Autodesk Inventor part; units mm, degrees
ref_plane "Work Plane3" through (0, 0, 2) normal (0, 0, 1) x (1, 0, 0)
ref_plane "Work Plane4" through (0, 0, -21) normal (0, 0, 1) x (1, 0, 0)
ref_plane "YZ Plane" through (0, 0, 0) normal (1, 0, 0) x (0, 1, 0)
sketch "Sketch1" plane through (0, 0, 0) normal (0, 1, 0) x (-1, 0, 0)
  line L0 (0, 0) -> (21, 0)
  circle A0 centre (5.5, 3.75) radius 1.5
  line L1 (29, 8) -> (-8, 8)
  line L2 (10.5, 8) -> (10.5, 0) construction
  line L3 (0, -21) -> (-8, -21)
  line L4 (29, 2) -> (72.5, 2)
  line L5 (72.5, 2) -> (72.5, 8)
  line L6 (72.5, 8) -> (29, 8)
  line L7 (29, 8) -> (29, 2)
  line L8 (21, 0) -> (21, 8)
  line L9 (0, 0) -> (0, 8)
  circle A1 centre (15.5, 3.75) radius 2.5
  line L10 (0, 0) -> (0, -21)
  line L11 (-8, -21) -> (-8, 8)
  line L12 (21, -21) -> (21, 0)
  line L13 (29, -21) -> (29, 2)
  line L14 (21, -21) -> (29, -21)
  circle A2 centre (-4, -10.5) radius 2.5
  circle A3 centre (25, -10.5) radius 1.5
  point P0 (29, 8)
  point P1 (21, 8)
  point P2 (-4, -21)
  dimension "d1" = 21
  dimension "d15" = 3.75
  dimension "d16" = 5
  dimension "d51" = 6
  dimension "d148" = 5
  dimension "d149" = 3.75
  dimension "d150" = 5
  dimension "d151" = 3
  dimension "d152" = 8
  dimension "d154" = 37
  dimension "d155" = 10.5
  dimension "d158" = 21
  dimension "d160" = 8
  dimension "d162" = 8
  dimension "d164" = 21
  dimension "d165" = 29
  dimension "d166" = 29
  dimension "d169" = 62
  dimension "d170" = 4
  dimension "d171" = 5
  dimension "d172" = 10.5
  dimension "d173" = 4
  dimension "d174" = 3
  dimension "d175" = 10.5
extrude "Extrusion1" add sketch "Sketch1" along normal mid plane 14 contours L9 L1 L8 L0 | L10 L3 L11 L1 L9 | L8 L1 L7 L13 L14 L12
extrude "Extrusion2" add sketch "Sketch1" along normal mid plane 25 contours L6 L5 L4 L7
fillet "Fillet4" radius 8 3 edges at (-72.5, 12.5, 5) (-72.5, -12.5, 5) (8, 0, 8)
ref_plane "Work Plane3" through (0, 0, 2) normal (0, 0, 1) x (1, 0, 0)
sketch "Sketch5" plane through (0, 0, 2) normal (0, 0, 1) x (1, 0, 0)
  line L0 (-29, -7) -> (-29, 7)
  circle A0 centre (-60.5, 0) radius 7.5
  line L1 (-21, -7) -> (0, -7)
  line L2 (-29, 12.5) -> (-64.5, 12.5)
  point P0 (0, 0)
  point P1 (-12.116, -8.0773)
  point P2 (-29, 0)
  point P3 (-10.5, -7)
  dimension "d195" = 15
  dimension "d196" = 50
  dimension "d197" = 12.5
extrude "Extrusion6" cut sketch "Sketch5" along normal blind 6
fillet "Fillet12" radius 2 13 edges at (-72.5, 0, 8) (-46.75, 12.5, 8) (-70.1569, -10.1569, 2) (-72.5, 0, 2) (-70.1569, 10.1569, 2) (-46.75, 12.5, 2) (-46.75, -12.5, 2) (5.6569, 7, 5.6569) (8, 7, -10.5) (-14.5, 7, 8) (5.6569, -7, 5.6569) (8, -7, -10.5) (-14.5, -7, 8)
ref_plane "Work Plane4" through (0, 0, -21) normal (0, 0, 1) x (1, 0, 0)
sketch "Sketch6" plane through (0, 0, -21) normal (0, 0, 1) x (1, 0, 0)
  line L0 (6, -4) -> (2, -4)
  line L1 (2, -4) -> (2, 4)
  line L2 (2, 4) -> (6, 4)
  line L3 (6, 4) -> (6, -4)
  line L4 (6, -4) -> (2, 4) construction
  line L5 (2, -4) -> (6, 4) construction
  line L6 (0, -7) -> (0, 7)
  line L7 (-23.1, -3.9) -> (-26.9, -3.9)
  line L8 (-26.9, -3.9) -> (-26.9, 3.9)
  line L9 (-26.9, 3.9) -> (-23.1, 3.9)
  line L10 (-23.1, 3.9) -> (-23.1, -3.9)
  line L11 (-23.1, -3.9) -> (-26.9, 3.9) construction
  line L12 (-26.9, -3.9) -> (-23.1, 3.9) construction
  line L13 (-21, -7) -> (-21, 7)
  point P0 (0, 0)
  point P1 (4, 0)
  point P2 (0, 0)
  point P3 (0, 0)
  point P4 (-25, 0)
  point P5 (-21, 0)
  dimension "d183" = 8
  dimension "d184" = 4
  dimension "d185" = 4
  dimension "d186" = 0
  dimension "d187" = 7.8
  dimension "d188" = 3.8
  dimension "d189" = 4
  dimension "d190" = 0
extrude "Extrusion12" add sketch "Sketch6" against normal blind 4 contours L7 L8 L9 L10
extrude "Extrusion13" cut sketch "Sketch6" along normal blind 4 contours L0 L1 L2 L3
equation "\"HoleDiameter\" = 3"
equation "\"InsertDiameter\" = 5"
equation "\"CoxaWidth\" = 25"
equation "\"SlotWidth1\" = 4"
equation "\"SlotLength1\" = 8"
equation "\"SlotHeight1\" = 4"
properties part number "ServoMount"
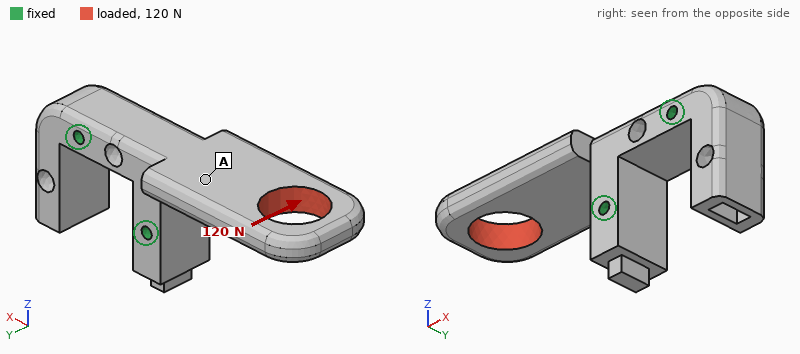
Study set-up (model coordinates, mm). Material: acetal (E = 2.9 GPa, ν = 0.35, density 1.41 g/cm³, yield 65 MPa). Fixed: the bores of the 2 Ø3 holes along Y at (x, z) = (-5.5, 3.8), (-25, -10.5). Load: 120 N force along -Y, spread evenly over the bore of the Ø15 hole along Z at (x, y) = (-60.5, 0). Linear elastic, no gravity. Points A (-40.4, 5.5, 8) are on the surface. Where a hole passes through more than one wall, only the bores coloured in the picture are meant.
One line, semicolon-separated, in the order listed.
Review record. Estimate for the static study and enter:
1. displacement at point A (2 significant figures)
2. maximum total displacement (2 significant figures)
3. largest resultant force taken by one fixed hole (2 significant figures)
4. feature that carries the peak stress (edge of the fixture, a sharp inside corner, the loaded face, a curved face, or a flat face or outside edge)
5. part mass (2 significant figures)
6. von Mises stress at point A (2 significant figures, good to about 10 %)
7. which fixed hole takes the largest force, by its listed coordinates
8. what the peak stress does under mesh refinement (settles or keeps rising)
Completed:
0.36 mm; 1.1 mm; 230 N; edge of the fixture; 18 g; 2.6 MPa; (-25, -10.5); keeps rising
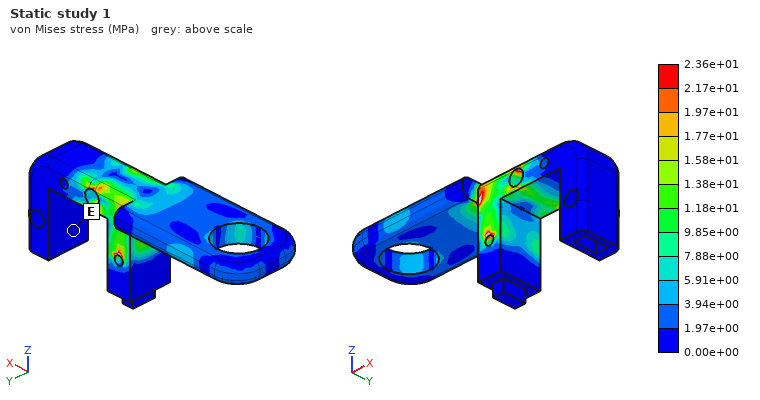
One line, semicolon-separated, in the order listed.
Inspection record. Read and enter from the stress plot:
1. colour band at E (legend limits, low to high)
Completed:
0.00e+00 to 1.97e+00 MPa
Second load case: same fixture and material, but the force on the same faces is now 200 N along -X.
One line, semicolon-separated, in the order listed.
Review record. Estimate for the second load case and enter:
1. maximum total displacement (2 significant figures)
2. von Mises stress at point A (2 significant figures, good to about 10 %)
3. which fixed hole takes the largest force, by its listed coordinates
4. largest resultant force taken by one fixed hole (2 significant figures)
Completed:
0.11 mm; 1.6 MPa; (-5.5, 3.8); 180 N
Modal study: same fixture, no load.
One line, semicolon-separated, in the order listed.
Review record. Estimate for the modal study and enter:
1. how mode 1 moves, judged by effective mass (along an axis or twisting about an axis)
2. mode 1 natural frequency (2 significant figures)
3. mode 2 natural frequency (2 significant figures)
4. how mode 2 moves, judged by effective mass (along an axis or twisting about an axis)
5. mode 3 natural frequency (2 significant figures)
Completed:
along Z; 650 Hz; 970 Hz; along Y; 1900 Hz
